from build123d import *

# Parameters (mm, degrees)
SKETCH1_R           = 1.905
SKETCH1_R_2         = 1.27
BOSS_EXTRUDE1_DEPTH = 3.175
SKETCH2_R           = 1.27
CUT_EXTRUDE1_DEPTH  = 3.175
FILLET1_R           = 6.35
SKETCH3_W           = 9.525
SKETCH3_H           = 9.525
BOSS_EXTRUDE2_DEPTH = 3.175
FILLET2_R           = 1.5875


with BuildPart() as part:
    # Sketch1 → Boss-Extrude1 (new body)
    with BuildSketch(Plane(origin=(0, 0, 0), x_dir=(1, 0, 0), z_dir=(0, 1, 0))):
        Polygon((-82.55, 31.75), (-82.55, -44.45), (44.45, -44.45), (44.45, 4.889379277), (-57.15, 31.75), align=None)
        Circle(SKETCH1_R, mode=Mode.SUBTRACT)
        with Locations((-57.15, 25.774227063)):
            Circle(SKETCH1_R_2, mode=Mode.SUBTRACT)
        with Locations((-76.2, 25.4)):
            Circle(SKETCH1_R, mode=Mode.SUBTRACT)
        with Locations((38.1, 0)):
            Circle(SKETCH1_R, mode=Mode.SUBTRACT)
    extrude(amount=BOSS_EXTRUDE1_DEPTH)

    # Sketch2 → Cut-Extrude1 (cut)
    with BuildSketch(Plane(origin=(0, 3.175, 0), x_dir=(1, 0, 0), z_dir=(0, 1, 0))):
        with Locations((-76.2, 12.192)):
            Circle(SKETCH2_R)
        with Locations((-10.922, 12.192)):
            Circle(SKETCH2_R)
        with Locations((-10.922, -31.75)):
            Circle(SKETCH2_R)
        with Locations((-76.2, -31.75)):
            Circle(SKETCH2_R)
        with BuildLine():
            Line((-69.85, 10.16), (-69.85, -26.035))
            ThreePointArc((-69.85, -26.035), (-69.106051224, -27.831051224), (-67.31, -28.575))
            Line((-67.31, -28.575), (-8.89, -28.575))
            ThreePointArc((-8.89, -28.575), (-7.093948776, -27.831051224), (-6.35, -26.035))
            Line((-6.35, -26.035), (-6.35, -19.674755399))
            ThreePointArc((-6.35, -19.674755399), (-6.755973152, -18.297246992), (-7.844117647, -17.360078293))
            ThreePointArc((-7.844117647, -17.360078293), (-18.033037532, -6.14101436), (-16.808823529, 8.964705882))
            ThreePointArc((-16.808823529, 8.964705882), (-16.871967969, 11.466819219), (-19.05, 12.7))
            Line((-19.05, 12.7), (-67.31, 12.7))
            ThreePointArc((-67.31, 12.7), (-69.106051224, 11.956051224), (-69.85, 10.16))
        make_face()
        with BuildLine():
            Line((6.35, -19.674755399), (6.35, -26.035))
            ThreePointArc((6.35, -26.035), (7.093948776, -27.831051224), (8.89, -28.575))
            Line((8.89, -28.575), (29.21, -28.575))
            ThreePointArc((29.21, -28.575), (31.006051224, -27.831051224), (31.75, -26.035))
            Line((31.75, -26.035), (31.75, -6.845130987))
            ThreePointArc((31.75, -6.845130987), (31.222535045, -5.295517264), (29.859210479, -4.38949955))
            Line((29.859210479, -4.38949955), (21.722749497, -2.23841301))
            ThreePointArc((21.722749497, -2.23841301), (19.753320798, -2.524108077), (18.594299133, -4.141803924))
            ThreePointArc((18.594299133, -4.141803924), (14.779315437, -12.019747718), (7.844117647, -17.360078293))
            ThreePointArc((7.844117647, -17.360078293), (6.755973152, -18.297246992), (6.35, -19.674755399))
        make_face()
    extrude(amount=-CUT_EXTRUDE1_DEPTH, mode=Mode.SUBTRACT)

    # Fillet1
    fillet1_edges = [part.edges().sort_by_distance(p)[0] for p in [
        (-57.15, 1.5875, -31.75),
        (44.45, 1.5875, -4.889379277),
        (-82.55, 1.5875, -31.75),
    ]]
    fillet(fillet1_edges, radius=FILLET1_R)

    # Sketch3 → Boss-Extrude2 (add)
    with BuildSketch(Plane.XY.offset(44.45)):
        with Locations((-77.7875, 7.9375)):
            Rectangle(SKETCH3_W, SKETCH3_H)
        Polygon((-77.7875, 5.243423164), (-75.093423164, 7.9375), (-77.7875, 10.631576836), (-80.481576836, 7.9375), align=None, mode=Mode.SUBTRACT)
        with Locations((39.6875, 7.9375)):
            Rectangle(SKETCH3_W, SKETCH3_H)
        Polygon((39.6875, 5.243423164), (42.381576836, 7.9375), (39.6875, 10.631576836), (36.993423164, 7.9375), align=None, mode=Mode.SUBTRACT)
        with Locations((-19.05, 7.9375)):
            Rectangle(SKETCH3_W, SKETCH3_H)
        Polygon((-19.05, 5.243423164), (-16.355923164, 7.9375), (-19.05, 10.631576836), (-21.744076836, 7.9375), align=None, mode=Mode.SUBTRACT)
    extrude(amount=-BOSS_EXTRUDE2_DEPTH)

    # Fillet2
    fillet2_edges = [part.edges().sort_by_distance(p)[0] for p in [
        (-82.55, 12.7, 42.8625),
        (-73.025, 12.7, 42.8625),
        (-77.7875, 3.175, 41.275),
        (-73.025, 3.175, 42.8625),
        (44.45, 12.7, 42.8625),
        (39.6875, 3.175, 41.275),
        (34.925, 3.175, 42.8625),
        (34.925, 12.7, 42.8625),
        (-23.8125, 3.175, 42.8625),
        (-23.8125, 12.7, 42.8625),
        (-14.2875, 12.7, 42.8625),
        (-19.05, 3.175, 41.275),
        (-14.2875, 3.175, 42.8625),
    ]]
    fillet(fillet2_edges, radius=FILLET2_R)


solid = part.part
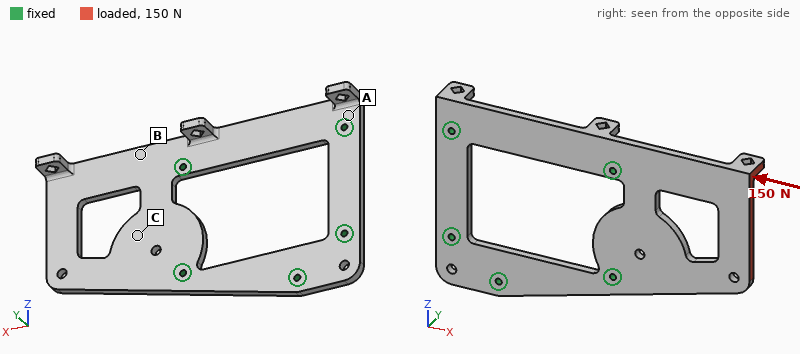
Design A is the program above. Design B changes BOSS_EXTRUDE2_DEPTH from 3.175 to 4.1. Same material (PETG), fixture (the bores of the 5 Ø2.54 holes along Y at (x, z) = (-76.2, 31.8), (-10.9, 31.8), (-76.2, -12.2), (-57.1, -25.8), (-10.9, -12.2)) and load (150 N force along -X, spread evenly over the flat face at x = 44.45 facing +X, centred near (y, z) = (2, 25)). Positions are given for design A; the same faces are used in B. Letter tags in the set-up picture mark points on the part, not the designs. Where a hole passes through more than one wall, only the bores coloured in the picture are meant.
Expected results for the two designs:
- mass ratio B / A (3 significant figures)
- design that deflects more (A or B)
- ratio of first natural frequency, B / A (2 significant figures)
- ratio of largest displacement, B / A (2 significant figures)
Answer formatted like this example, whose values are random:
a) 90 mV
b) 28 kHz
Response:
a) 1.01
b) B
c) 0.99
d) 1.2
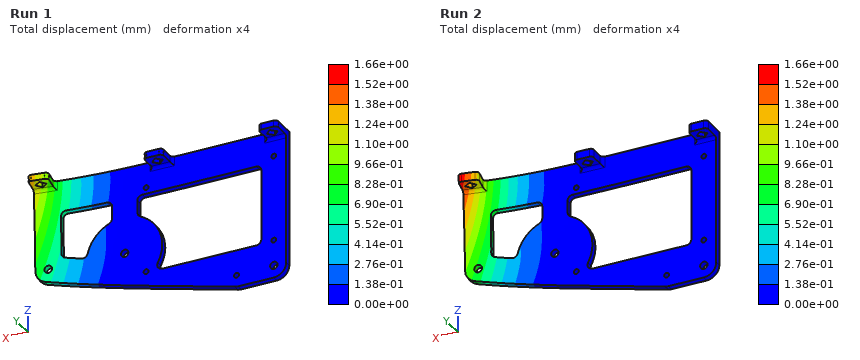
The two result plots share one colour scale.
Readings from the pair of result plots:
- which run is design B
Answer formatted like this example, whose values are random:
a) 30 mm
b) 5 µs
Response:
a) Run 2
